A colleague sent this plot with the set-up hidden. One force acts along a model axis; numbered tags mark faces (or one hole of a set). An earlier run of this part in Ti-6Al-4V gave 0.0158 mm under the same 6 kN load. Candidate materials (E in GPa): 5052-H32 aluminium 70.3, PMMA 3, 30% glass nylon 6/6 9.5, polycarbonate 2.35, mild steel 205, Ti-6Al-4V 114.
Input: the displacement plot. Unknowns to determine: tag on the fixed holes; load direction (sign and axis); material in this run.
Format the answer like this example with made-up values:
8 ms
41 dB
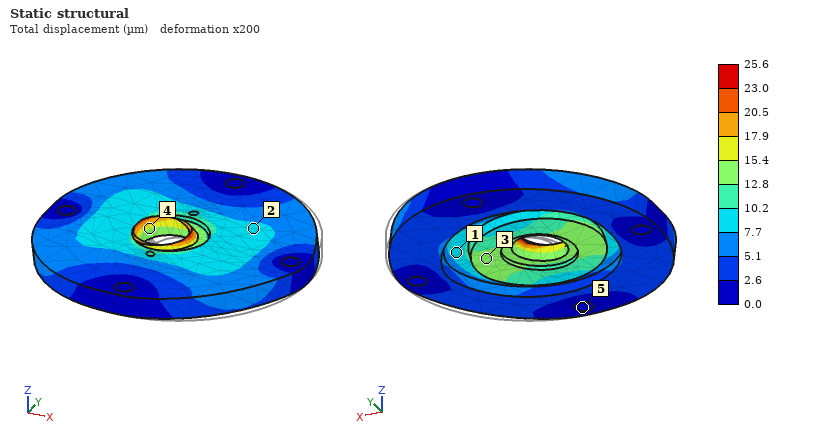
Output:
5
-X
5052-H32 aluminium
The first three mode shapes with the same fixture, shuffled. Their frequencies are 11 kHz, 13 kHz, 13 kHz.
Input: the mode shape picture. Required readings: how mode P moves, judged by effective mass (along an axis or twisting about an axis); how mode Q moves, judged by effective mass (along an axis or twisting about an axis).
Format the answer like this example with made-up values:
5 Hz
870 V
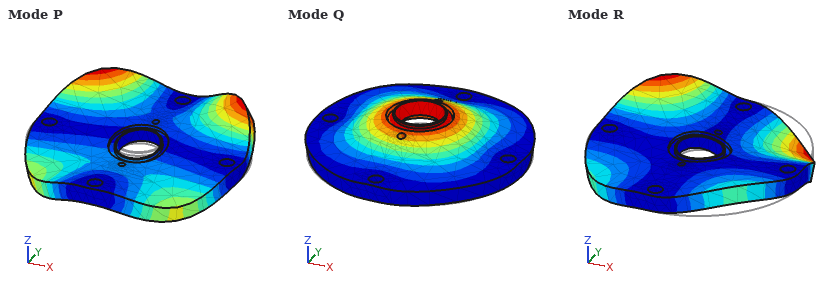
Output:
twisting about X
along Z
